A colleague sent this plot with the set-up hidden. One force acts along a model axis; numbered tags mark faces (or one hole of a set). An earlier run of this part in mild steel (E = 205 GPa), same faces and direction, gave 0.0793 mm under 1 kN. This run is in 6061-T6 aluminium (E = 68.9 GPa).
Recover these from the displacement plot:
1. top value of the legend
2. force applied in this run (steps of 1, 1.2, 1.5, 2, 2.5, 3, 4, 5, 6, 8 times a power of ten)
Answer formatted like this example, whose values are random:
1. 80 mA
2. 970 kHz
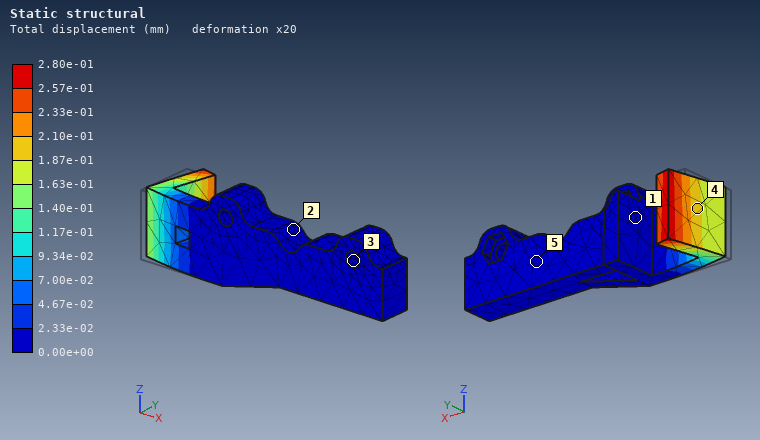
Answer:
1. 2.80e-01 mm
2. 1.2 kN
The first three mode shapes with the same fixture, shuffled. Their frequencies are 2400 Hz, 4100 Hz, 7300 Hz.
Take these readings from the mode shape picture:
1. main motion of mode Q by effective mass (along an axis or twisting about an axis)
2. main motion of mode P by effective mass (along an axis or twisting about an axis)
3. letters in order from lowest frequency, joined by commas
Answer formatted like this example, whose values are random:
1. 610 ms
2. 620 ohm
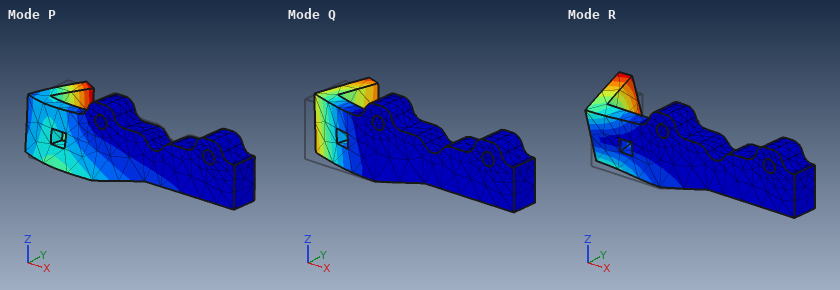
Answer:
1. along Y
2. along Y
3. Q, R, P
